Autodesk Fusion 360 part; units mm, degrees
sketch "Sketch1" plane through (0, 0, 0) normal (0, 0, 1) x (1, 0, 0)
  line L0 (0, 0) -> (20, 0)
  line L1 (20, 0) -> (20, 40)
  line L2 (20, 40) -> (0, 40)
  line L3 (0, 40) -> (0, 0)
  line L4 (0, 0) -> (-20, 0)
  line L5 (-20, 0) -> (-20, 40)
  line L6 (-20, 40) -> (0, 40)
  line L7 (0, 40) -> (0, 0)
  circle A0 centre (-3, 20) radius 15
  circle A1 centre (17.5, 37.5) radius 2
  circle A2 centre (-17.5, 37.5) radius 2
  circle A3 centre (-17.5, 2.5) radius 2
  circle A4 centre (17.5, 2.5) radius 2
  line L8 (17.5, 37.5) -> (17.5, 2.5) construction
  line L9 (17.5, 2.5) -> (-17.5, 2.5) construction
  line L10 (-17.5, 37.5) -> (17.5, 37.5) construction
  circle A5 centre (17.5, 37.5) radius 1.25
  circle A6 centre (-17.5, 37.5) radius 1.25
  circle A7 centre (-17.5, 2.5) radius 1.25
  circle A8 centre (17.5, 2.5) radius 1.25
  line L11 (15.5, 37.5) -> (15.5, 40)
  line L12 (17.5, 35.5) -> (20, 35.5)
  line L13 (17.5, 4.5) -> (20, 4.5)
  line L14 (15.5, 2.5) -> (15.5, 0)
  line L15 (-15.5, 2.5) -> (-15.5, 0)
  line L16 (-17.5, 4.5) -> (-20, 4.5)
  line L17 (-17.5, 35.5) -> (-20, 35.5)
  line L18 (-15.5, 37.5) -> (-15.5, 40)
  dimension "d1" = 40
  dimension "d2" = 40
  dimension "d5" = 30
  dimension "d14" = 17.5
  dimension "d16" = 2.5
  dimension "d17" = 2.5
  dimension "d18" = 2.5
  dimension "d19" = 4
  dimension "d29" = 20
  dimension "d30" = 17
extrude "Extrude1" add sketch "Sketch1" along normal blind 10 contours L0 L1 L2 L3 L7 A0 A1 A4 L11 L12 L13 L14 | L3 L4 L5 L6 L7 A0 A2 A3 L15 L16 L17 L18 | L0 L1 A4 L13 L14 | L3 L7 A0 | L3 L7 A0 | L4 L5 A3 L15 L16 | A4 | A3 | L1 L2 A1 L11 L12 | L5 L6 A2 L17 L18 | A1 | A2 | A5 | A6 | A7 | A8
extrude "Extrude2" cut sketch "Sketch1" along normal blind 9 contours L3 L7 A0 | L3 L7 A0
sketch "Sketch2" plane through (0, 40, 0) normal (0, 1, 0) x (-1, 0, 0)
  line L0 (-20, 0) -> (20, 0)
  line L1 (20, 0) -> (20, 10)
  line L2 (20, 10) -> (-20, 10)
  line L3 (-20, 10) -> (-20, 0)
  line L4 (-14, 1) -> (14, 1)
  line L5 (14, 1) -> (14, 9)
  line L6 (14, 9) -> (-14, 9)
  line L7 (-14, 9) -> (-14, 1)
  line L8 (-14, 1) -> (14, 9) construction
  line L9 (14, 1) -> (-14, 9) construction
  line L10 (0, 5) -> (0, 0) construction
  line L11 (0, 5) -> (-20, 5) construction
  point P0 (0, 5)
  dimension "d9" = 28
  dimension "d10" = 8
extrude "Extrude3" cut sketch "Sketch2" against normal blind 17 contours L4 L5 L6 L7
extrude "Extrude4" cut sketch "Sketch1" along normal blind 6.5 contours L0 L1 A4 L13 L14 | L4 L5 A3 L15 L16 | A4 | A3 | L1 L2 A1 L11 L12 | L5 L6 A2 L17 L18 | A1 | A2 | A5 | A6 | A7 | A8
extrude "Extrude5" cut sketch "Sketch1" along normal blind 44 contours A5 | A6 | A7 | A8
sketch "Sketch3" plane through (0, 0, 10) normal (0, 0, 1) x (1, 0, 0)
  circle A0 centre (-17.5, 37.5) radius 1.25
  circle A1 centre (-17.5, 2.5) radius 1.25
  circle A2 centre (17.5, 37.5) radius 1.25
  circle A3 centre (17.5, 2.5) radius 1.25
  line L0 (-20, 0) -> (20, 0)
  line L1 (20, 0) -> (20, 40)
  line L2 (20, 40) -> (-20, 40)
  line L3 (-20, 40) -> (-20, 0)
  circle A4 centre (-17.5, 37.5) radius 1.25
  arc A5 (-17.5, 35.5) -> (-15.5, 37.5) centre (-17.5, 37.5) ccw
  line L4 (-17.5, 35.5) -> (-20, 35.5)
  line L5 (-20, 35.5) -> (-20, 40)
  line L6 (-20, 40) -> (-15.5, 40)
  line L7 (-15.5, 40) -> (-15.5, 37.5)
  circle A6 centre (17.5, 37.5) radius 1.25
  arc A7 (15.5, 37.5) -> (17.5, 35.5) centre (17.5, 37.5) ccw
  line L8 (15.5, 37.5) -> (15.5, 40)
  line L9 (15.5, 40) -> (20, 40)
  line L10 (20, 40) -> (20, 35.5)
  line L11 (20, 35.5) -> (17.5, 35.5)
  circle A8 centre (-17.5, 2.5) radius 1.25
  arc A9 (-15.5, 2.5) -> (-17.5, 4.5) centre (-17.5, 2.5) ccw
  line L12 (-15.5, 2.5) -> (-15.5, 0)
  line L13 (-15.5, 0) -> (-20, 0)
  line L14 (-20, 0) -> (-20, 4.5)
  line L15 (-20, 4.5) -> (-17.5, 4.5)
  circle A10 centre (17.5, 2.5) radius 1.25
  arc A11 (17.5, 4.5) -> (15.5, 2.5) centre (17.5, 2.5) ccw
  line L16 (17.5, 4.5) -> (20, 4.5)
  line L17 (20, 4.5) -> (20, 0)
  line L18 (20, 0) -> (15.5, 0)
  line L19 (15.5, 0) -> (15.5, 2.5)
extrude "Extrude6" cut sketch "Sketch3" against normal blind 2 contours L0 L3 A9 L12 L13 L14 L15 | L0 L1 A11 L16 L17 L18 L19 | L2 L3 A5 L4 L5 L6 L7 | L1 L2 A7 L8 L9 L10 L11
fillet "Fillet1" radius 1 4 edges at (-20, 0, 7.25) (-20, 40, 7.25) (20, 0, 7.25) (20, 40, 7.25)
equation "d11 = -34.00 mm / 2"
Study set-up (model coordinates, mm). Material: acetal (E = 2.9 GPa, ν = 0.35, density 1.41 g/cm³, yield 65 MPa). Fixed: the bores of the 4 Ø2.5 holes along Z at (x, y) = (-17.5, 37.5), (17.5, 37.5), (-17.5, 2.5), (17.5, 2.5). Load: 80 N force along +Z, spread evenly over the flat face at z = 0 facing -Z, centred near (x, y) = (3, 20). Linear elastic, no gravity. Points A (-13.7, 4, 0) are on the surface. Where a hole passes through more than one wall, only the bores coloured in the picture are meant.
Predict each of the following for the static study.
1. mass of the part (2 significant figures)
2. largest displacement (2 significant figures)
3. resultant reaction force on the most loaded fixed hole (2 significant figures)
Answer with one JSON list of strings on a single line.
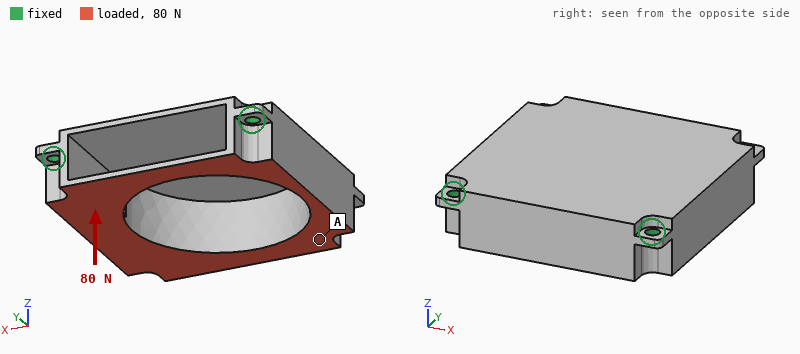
["10 g", "0.68 mm", "25 N"]
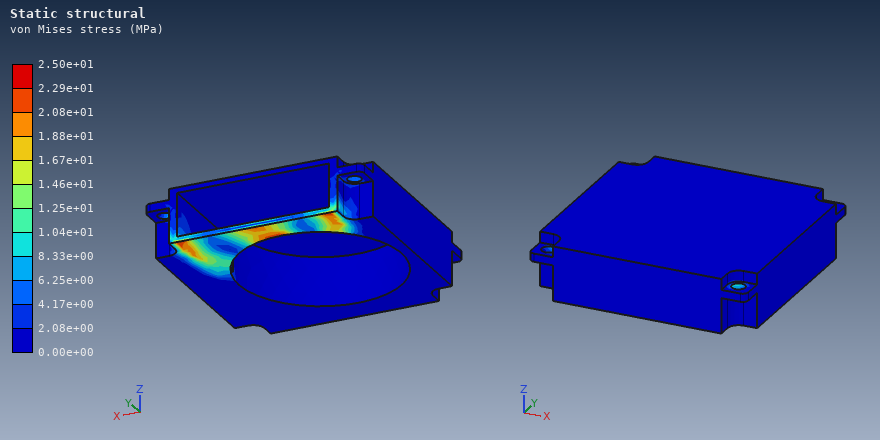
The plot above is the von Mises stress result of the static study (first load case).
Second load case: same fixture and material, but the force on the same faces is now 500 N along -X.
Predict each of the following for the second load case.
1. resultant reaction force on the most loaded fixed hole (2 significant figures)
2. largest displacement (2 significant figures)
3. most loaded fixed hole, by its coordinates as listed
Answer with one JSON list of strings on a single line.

["170 N", "0.35 mm", "(-17.5, 2.5)"]
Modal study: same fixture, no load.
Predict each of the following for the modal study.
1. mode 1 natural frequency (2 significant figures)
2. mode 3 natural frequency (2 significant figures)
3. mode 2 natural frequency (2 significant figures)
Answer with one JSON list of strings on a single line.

["1900 Hz", "2700 Hz", "2000 Hz"]
